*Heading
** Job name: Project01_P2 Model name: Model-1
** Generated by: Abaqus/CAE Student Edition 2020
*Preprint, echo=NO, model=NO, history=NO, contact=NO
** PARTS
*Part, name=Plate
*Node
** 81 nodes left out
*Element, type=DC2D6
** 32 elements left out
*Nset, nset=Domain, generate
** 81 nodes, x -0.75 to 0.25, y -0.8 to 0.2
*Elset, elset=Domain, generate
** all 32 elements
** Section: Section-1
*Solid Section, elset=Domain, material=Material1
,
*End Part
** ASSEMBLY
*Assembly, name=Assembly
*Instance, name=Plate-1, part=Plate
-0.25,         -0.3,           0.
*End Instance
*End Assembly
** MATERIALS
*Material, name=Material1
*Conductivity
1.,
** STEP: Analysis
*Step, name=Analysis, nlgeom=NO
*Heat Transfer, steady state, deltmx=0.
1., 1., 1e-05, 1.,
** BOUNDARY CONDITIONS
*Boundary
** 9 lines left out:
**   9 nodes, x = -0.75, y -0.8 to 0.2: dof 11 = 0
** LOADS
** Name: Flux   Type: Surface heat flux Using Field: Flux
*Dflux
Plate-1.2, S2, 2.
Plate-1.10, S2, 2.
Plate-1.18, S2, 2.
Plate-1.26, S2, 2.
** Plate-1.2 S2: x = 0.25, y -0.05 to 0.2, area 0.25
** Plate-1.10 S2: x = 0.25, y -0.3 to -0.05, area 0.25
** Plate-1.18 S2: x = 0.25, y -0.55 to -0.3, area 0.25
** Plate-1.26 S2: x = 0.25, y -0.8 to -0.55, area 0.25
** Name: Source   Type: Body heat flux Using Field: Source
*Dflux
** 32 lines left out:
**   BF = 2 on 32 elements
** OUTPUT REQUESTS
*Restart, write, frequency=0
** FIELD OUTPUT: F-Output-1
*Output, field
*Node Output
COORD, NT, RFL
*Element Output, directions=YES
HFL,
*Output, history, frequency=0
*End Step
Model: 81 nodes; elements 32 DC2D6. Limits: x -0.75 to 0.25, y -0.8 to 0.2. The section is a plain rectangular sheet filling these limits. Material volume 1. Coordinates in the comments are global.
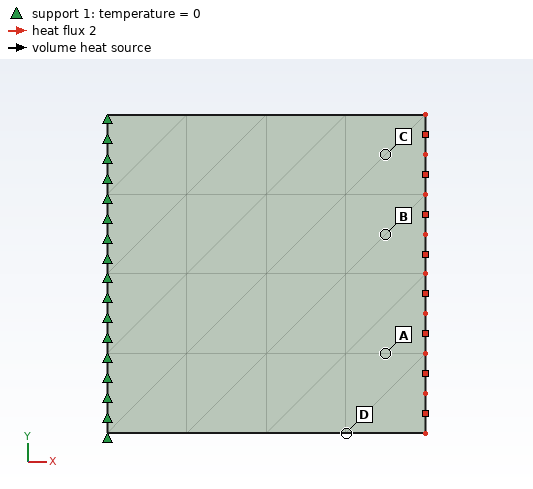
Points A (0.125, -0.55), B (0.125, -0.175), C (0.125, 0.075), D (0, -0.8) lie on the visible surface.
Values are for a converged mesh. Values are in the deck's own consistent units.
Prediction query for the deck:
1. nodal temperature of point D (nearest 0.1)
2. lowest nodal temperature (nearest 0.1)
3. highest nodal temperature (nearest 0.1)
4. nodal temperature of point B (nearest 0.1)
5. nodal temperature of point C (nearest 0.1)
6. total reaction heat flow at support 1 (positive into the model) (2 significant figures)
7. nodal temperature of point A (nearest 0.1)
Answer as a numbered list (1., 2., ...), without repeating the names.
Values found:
1. 2.4
2. 0.0
3. 3.0
4. 2.7
5. 2.7
6. -4.0
7. 2.7
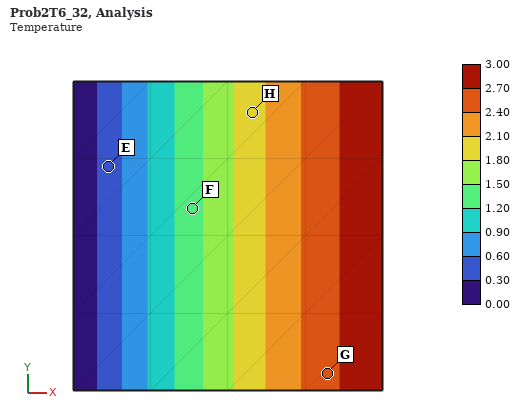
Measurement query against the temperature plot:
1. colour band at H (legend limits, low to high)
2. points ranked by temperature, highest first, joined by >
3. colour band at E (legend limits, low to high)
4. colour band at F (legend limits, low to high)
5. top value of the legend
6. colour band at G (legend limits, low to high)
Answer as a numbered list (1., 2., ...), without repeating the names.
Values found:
1. 1.80 to 2.10
2. G > H > F > E
3. 0.30 to 0.60
4. 1.20 to 1.50
5. 3.00
6. 2.40 to 2.70
